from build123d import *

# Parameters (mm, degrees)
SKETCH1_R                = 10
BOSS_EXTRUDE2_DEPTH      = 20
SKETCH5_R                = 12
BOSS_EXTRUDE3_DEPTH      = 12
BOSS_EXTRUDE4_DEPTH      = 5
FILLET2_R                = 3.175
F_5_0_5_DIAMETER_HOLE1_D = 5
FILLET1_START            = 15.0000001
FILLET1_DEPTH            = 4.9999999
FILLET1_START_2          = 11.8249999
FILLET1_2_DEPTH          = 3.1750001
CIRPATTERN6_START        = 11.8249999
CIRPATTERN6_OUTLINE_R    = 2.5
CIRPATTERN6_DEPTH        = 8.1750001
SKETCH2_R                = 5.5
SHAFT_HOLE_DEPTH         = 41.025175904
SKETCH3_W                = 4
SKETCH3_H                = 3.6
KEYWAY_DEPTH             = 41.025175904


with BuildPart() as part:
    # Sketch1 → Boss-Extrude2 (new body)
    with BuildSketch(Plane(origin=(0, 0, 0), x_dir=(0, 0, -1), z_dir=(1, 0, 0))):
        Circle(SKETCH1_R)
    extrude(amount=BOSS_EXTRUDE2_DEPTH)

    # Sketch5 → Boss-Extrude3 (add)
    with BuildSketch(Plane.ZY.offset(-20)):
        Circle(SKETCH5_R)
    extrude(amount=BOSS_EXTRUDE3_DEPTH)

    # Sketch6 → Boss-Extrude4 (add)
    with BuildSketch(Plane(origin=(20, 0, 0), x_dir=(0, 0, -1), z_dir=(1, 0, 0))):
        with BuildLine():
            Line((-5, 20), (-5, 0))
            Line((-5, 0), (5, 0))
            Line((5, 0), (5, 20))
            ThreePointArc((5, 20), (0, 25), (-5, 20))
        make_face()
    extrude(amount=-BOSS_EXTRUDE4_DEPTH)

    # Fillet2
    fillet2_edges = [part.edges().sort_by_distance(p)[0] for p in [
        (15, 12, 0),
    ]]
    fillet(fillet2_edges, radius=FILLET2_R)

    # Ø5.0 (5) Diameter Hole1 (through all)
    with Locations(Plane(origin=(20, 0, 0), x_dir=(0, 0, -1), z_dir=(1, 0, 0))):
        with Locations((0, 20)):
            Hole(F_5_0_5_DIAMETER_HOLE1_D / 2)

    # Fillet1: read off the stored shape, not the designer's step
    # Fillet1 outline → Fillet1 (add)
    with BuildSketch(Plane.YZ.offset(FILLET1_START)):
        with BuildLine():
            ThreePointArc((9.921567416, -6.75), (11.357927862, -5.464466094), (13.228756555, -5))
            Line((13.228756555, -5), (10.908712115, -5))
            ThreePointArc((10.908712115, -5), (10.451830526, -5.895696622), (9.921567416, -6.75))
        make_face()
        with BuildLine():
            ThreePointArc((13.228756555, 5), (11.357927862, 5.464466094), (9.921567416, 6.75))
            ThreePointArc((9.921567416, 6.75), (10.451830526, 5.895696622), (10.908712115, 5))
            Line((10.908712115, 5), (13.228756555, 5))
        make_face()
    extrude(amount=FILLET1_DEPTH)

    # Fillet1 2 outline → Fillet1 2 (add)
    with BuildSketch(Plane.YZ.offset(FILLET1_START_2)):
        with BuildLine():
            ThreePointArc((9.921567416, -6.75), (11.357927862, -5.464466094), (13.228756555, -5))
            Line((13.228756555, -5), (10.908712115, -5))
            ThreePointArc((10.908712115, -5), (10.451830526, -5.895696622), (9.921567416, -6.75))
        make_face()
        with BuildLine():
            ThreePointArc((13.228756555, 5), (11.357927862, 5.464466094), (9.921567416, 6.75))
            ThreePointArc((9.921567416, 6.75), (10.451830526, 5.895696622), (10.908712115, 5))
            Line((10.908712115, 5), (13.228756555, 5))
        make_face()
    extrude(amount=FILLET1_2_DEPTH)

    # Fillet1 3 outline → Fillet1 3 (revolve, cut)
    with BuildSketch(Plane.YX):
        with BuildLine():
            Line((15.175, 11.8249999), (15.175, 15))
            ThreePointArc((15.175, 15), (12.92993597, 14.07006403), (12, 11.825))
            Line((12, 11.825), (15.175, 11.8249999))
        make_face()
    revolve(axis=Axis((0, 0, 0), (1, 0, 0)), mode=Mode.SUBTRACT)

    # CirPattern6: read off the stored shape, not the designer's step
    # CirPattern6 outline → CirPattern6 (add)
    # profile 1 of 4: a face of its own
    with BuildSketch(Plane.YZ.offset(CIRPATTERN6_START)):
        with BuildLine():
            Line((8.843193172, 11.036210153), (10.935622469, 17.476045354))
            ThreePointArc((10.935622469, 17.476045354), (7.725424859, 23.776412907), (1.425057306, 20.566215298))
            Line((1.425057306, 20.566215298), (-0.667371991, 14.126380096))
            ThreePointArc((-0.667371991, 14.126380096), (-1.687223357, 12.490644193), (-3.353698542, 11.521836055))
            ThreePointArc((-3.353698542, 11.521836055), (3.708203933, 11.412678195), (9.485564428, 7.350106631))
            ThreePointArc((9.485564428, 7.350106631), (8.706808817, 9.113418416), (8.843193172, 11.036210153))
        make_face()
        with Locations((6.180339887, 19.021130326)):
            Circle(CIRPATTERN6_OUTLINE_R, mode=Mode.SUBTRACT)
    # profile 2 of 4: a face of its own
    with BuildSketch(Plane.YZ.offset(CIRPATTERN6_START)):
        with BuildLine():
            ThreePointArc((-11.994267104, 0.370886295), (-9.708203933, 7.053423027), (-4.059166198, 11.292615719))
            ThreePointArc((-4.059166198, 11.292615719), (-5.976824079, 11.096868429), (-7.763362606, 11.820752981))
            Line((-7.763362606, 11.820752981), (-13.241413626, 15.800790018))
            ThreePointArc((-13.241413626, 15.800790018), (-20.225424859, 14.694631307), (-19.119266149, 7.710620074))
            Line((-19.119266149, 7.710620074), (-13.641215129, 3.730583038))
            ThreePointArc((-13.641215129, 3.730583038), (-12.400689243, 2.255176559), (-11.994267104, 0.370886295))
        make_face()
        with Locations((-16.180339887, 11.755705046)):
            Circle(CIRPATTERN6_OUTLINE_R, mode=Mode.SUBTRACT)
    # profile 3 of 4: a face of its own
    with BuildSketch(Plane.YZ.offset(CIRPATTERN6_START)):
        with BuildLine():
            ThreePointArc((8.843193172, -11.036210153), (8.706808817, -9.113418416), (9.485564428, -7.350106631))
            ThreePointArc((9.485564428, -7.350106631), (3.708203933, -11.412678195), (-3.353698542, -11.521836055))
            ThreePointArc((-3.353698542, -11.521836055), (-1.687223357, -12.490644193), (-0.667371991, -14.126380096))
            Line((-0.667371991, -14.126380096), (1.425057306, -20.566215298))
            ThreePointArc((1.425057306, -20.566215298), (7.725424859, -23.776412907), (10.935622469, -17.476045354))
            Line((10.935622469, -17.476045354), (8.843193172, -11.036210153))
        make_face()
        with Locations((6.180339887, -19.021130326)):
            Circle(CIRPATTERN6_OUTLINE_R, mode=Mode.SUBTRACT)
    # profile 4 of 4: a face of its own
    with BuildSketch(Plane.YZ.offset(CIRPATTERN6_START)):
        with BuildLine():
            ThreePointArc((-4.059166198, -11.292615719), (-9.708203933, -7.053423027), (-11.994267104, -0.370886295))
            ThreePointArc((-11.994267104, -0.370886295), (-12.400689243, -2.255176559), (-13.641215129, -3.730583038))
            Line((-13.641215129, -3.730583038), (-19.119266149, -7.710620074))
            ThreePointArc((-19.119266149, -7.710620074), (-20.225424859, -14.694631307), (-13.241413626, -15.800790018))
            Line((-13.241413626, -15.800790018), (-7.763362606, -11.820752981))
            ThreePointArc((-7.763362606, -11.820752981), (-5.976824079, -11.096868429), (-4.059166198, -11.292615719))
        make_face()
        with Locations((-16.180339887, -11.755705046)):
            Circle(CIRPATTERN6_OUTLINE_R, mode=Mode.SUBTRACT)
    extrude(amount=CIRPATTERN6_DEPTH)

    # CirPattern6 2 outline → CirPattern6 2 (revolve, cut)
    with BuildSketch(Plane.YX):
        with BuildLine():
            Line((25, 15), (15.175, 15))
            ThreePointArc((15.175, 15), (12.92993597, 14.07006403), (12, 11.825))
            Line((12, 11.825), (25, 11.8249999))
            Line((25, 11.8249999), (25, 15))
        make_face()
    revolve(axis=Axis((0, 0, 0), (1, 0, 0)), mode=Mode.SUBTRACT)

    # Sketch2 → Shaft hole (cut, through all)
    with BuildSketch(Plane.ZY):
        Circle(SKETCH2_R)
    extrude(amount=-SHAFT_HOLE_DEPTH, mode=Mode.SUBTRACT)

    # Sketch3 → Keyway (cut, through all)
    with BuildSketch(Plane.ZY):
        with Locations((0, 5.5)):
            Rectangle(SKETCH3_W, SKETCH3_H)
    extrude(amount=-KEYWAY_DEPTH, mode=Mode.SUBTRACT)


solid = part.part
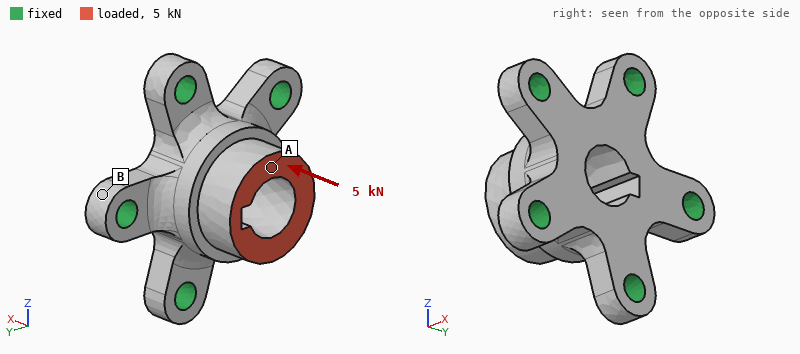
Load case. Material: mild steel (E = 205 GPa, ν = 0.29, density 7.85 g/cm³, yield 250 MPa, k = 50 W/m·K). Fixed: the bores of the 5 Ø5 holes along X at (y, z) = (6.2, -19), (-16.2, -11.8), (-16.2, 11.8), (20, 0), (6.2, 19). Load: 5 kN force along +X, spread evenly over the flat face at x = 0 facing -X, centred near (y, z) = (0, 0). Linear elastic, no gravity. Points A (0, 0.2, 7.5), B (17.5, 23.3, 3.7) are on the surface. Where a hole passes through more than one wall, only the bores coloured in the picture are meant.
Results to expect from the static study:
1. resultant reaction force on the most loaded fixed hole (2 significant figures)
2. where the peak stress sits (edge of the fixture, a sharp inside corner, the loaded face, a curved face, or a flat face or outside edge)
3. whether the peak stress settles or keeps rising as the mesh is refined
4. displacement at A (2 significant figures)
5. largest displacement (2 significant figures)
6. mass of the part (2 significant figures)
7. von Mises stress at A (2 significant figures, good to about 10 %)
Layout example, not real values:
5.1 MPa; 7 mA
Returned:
1.2 kN; edge of the fixture; keeps rising; 5.4 µm; 5.7 µm; 68 g; 24 MPa
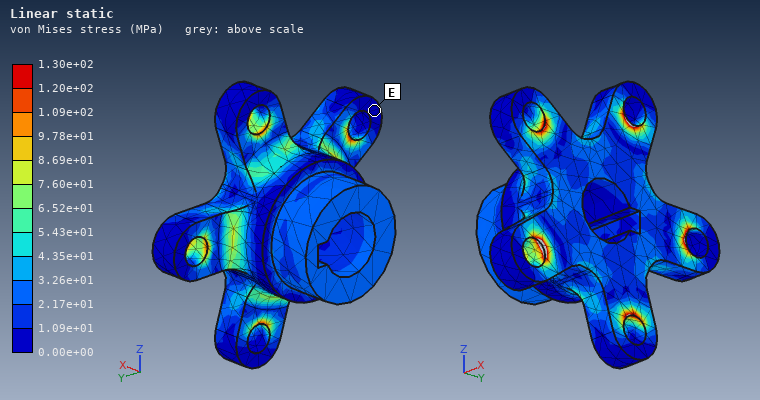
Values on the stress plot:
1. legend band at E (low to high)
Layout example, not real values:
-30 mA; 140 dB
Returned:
0.00e+00 to 1.09e+01 MPa
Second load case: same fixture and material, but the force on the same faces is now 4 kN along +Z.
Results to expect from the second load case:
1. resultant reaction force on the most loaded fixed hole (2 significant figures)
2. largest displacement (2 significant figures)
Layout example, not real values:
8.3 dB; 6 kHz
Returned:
2.1 kN; 17 µm
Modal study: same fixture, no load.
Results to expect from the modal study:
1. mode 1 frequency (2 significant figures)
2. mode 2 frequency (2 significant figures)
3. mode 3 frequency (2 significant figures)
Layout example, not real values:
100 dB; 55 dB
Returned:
24 kHz; 24 kHz; 24 kHz
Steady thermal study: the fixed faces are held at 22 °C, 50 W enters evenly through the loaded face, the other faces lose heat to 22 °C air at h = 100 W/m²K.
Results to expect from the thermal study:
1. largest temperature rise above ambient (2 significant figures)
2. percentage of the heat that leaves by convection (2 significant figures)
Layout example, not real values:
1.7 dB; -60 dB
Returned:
82 K; 22 %
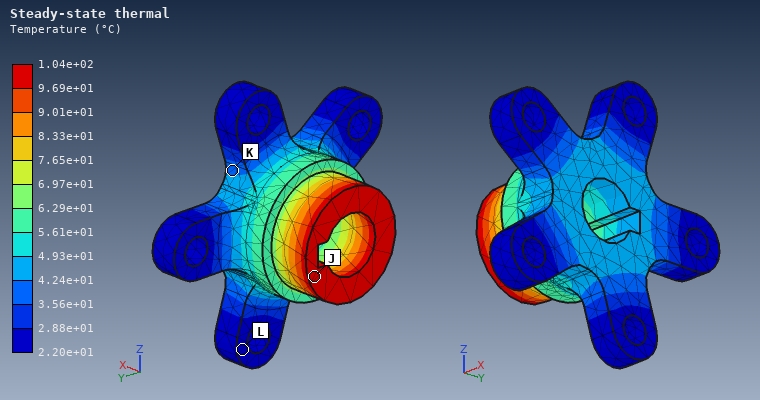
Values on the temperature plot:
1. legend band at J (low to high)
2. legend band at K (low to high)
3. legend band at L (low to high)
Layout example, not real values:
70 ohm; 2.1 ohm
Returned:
9.69e+01 to 1.04e+02 °C; 3.56e+01 to 4.24e+01 °C; 2.20e+01 to 2.88e+01 °C
